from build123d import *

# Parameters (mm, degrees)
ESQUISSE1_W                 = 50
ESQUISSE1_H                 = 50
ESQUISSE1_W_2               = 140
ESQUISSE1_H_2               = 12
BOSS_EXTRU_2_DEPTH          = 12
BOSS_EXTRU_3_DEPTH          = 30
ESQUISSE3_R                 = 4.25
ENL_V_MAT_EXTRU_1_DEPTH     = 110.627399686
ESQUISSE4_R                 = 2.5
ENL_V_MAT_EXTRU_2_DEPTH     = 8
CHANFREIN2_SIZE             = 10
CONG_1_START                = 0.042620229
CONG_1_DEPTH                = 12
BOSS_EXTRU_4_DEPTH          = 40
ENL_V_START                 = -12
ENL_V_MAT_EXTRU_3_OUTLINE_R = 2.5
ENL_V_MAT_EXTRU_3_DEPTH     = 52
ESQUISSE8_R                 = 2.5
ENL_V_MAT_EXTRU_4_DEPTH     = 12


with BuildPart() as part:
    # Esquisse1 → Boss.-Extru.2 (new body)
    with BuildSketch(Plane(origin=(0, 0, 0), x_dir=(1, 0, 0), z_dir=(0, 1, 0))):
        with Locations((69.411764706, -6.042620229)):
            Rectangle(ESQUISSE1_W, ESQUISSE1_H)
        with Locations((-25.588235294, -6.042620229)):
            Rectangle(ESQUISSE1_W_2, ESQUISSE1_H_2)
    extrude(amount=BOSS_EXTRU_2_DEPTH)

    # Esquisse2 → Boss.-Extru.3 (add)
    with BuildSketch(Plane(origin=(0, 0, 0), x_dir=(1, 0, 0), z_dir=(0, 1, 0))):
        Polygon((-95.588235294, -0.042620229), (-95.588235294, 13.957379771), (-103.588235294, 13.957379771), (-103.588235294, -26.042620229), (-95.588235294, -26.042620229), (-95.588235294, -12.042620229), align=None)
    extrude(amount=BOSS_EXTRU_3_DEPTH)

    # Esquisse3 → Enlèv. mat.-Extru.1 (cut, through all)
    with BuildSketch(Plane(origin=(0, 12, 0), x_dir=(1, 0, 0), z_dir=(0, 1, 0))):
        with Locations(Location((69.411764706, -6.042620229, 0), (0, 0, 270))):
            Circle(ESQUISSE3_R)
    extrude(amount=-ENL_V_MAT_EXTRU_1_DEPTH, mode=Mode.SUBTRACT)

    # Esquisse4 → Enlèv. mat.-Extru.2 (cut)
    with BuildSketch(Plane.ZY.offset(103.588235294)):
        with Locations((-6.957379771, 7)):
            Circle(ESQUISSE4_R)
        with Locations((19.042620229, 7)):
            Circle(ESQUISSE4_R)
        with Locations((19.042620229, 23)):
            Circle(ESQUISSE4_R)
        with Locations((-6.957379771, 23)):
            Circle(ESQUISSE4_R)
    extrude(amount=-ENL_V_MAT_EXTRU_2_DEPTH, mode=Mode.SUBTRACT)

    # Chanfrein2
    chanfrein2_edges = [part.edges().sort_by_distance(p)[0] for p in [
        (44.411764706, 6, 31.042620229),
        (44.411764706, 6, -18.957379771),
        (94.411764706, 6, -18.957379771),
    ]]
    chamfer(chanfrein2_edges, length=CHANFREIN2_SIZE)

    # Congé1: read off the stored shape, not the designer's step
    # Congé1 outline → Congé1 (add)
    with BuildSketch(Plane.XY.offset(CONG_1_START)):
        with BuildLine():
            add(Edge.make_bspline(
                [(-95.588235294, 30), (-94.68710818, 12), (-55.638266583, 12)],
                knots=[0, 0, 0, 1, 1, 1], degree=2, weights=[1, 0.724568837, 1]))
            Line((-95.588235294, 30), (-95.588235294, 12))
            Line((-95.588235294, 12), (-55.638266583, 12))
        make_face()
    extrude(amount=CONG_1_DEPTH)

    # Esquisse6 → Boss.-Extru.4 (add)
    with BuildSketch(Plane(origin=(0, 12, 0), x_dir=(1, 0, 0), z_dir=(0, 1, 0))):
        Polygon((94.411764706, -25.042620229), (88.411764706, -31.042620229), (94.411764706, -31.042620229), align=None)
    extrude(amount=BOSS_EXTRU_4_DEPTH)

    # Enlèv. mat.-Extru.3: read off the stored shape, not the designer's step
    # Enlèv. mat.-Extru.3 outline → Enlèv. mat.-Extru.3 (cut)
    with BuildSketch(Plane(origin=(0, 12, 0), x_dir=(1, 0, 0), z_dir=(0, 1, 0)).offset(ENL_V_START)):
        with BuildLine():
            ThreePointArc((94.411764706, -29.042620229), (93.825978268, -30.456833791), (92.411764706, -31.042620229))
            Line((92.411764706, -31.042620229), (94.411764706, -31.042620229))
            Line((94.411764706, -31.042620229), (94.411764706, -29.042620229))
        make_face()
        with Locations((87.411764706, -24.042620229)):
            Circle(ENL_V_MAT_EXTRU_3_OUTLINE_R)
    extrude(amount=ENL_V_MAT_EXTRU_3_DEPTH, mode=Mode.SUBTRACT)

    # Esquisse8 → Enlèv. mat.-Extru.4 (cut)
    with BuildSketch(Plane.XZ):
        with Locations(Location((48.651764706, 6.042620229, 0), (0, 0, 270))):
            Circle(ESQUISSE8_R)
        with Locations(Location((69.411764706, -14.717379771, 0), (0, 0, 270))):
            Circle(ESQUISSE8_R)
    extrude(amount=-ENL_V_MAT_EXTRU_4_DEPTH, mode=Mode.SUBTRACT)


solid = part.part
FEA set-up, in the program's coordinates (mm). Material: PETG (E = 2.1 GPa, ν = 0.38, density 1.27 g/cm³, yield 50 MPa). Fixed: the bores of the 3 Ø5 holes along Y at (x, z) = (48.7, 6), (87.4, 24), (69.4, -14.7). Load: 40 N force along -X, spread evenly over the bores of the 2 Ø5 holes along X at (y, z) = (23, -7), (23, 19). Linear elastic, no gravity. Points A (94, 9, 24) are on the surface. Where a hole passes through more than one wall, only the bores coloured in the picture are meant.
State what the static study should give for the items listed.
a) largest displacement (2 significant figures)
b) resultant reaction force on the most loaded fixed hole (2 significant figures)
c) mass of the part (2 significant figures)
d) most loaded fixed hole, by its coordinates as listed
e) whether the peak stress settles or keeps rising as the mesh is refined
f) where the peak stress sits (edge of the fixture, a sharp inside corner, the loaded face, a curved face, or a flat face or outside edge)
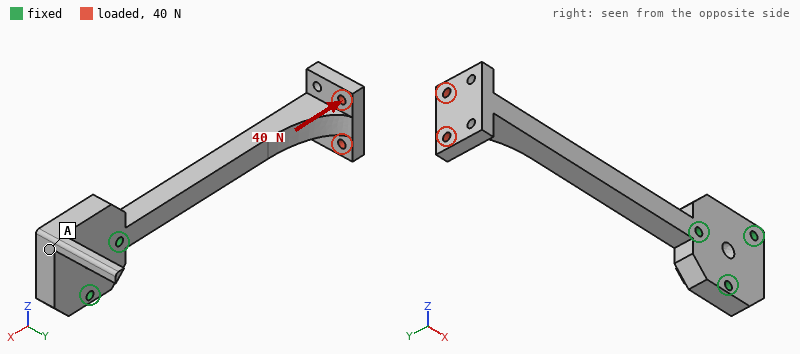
2.1 mm
36 N
74 g
(48.7, 6)
keeps rising
edge of the fixture
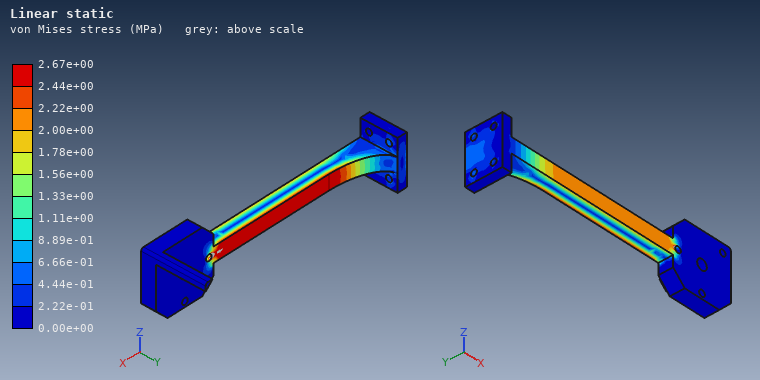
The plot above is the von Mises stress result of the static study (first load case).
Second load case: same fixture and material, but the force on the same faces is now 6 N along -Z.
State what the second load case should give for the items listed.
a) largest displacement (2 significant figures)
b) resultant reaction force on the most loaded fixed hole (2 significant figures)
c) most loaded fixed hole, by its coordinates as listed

2.0 mm
18 N
(69.4, -14.7)
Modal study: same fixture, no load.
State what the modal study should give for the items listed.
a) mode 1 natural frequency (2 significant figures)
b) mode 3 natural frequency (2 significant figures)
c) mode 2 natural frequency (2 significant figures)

67 Hz
370 Hz
68 Hz
